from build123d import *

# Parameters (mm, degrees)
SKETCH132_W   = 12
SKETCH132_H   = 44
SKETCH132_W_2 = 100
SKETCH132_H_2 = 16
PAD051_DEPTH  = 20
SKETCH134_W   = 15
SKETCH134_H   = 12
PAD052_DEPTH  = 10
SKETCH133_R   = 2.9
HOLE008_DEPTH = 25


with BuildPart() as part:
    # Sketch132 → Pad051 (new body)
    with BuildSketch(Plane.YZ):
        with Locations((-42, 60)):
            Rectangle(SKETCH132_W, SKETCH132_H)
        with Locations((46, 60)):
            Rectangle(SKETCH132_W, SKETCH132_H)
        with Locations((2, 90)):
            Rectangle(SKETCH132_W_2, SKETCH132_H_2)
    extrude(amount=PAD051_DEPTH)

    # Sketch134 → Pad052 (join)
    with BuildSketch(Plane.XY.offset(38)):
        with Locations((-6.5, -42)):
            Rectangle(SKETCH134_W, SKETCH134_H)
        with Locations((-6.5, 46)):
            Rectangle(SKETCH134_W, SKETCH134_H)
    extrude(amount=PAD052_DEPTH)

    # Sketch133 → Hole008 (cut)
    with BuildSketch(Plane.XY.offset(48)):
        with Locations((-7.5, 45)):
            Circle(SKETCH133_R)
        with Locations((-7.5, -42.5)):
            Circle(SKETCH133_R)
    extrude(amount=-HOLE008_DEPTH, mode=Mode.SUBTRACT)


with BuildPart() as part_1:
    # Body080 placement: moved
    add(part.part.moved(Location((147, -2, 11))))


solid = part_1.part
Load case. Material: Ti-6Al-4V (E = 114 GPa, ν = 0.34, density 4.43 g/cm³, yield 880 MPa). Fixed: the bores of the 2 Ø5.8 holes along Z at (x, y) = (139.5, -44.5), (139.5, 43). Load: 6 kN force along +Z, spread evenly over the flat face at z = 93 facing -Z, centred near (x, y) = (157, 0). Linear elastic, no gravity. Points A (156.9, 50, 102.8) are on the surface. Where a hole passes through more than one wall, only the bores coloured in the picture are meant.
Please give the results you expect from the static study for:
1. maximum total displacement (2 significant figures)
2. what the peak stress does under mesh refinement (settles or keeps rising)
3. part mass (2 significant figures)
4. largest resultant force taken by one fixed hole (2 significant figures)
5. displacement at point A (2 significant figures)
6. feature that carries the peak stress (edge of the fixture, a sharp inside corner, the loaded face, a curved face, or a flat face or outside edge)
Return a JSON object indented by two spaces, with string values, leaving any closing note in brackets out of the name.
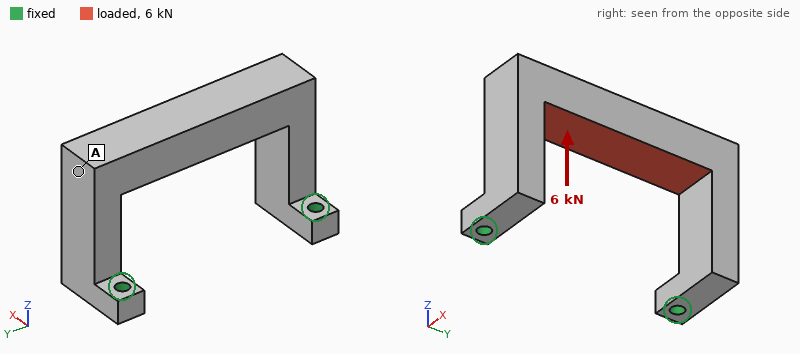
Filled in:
{
  "maximum total displacement": "0.22 mm",
  "what the peak stress does under mesh refinement": "keeps rising",
  "part mass": "250 g",
  "largest resultant force taken by one fixed hole": "3.1 kN",
  "displacement at point A": "0.16 mm",
  "feature that carries the peak stress": "edge of the fixture"
}
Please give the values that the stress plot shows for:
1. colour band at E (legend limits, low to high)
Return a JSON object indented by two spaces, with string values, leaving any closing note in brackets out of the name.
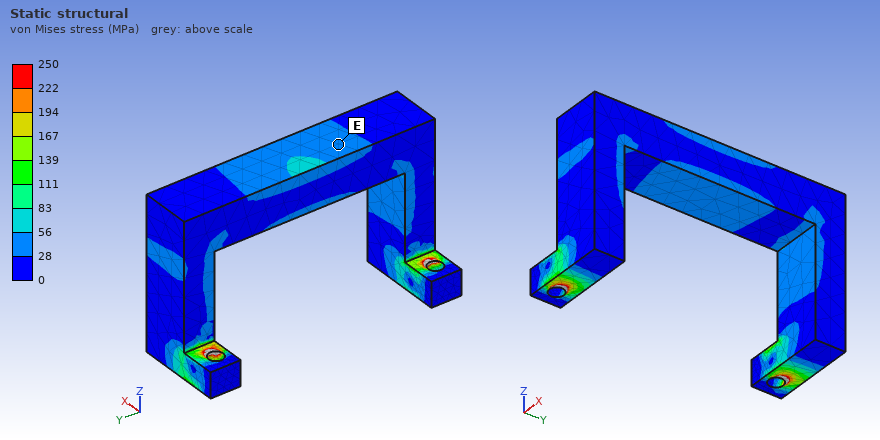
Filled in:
{
  "colour band at E": "28 to 56 MPa"
}
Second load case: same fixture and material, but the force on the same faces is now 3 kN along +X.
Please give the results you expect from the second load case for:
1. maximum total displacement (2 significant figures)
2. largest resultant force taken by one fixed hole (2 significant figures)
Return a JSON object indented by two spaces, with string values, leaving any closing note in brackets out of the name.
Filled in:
{
  "maximum total displacement": "0.40 mm",
  "largest resultant force taken by one fixed hole": "1.5 kN"
}
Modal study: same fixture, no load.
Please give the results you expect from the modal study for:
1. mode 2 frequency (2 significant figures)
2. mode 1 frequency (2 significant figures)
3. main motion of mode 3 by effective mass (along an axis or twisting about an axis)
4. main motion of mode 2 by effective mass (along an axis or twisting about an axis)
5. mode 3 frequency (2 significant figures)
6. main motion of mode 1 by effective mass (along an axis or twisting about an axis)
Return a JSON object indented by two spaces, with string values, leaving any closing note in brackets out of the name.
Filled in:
{
  "mode 2 frequency": "1900 Hz",
  "mode 1 frequency": "1100 Hz",
  "main motion of mode 3 by effective mass": "twisting about Z",
  "main motion of mode 2 by effective mass": "along Y",
  "mode 3 frequency": "2600 Hz",
  "main motion of mode 1 by effective mass": "along X"
}
